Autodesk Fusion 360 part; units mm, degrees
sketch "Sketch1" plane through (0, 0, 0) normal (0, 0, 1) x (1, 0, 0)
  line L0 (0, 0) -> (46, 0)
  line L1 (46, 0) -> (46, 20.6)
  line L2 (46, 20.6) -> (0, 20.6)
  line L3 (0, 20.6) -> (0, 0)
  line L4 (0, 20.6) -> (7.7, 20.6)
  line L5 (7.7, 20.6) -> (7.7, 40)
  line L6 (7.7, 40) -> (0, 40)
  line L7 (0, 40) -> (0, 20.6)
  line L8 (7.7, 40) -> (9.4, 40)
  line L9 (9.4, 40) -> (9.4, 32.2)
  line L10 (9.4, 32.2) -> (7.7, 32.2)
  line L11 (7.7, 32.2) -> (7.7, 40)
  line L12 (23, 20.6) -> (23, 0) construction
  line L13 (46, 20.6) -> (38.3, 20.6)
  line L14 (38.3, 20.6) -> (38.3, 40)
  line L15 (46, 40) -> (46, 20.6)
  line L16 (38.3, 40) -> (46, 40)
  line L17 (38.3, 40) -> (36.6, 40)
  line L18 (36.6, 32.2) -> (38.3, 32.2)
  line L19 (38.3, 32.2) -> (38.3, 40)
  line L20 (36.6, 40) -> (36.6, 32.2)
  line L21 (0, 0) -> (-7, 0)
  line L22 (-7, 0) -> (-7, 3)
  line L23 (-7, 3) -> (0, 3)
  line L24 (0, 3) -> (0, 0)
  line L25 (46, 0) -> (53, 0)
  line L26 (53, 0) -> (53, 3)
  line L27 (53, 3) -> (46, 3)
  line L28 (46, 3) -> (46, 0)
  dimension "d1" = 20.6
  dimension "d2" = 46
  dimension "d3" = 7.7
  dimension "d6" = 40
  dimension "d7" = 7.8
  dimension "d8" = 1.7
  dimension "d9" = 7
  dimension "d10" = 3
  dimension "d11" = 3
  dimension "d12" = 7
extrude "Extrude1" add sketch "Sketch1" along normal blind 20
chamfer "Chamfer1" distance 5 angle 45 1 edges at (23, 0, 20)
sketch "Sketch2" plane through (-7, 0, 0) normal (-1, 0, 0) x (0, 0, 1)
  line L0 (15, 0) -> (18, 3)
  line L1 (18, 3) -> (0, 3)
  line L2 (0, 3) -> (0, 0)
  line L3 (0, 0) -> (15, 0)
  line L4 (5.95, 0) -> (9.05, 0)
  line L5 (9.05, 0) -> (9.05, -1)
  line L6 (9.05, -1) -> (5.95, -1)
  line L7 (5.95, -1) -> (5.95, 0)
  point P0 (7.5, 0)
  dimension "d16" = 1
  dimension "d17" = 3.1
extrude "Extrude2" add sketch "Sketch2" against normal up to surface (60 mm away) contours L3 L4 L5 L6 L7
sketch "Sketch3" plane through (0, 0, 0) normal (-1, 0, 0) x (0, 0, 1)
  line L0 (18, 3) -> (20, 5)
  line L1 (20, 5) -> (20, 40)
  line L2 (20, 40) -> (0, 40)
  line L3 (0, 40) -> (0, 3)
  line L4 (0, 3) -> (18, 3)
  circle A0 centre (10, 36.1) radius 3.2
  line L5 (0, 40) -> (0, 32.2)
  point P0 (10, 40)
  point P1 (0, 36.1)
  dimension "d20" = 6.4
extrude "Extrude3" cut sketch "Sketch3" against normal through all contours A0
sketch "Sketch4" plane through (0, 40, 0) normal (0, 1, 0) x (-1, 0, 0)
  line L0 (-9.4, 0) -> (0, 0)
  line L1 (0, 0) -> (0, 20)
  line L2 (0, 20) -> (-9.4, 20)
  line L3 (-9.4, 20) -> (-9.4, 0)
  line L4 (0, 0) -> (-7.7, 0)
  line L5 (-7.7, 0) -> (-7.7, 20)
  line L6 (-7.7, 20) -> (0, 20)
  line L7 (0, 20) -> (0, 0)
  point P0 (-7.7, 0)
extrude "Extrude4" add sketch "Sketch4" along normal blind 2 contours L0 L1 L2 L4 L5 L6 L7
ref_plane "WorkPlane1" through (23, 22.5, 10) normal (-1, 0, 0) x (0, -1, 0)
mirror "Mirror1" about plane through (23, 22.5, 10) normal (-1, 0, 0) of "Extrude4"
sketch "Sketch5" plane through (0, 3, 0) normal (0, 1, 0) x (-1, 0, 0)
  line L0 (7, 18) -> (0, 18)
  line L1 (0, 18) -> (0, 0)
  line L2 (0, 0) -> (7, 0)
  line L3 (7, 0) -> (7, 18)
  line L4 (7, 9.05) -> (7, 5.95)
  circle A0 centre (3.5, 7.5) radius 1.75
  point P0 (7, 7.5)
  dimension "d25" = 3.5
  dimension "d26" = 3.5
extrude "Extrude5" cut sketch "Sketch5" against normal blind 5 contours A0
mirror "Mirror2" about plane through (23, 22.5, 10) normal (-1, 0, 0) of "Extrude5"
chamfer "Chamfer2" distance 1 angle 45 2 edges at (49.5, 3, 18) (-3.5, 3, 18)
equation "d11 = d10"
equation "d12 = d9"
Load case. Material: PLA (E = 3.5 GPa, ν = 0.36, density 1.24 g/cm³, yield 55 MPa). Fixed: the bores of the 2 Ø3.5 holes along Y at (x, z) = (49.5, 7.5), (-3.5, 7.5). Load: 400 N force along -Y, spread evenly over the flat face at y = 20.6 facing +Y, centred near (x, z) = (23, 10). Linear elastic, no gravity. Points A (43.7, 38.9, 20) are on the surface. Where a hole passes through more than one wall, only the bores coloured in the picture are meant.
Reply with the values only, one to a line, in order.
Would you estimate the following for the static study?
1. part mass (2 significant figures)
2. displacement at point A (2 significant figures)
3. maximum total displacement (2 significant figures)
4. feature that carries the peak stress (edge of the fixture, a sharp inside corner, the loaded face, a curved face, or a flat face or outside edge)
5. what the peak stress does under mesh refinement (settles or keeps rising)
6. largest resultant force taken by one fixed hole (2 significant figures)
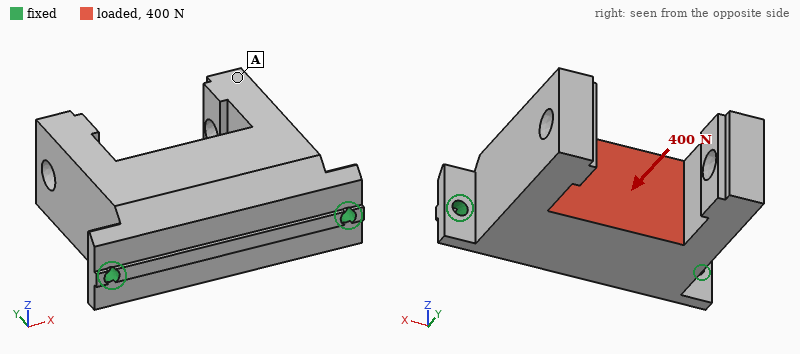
32 g
0.35 mm
0.37 mm
edge of the fixture
keeps rising
240 N
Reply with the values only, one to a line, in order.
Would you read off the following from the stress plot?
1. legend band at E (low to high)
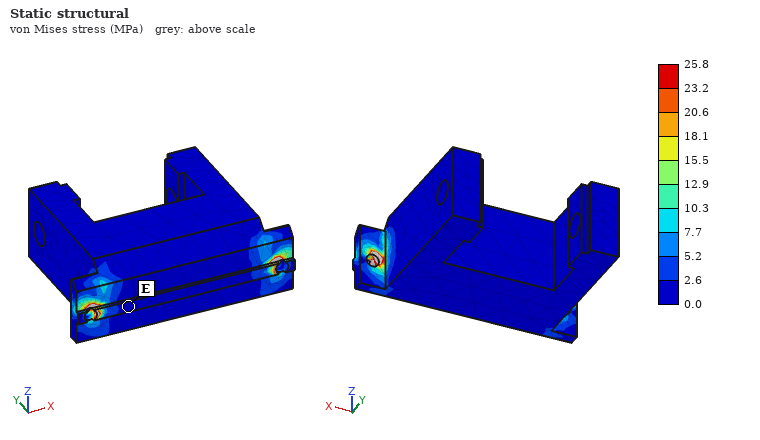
0.0 to 2.6 MPa
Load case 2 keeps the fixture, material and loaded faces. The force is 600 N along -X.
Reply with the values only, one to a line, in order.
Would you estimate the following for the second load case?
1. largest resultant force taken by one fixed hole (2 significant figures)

390 N
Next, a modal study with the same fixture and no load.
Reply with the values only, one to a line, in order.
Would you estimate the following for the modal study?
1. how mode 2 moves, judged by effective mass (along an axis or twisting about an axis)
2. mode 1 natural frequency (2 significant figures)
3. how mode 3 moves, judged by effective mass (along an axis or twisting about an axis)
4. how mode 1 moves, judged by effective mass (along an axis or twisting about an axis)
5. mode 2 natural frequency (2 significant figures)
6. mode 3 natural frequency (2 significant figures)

along X
500 Hz
twisting about Y
along Z
2300 Hz
2700 Hz
